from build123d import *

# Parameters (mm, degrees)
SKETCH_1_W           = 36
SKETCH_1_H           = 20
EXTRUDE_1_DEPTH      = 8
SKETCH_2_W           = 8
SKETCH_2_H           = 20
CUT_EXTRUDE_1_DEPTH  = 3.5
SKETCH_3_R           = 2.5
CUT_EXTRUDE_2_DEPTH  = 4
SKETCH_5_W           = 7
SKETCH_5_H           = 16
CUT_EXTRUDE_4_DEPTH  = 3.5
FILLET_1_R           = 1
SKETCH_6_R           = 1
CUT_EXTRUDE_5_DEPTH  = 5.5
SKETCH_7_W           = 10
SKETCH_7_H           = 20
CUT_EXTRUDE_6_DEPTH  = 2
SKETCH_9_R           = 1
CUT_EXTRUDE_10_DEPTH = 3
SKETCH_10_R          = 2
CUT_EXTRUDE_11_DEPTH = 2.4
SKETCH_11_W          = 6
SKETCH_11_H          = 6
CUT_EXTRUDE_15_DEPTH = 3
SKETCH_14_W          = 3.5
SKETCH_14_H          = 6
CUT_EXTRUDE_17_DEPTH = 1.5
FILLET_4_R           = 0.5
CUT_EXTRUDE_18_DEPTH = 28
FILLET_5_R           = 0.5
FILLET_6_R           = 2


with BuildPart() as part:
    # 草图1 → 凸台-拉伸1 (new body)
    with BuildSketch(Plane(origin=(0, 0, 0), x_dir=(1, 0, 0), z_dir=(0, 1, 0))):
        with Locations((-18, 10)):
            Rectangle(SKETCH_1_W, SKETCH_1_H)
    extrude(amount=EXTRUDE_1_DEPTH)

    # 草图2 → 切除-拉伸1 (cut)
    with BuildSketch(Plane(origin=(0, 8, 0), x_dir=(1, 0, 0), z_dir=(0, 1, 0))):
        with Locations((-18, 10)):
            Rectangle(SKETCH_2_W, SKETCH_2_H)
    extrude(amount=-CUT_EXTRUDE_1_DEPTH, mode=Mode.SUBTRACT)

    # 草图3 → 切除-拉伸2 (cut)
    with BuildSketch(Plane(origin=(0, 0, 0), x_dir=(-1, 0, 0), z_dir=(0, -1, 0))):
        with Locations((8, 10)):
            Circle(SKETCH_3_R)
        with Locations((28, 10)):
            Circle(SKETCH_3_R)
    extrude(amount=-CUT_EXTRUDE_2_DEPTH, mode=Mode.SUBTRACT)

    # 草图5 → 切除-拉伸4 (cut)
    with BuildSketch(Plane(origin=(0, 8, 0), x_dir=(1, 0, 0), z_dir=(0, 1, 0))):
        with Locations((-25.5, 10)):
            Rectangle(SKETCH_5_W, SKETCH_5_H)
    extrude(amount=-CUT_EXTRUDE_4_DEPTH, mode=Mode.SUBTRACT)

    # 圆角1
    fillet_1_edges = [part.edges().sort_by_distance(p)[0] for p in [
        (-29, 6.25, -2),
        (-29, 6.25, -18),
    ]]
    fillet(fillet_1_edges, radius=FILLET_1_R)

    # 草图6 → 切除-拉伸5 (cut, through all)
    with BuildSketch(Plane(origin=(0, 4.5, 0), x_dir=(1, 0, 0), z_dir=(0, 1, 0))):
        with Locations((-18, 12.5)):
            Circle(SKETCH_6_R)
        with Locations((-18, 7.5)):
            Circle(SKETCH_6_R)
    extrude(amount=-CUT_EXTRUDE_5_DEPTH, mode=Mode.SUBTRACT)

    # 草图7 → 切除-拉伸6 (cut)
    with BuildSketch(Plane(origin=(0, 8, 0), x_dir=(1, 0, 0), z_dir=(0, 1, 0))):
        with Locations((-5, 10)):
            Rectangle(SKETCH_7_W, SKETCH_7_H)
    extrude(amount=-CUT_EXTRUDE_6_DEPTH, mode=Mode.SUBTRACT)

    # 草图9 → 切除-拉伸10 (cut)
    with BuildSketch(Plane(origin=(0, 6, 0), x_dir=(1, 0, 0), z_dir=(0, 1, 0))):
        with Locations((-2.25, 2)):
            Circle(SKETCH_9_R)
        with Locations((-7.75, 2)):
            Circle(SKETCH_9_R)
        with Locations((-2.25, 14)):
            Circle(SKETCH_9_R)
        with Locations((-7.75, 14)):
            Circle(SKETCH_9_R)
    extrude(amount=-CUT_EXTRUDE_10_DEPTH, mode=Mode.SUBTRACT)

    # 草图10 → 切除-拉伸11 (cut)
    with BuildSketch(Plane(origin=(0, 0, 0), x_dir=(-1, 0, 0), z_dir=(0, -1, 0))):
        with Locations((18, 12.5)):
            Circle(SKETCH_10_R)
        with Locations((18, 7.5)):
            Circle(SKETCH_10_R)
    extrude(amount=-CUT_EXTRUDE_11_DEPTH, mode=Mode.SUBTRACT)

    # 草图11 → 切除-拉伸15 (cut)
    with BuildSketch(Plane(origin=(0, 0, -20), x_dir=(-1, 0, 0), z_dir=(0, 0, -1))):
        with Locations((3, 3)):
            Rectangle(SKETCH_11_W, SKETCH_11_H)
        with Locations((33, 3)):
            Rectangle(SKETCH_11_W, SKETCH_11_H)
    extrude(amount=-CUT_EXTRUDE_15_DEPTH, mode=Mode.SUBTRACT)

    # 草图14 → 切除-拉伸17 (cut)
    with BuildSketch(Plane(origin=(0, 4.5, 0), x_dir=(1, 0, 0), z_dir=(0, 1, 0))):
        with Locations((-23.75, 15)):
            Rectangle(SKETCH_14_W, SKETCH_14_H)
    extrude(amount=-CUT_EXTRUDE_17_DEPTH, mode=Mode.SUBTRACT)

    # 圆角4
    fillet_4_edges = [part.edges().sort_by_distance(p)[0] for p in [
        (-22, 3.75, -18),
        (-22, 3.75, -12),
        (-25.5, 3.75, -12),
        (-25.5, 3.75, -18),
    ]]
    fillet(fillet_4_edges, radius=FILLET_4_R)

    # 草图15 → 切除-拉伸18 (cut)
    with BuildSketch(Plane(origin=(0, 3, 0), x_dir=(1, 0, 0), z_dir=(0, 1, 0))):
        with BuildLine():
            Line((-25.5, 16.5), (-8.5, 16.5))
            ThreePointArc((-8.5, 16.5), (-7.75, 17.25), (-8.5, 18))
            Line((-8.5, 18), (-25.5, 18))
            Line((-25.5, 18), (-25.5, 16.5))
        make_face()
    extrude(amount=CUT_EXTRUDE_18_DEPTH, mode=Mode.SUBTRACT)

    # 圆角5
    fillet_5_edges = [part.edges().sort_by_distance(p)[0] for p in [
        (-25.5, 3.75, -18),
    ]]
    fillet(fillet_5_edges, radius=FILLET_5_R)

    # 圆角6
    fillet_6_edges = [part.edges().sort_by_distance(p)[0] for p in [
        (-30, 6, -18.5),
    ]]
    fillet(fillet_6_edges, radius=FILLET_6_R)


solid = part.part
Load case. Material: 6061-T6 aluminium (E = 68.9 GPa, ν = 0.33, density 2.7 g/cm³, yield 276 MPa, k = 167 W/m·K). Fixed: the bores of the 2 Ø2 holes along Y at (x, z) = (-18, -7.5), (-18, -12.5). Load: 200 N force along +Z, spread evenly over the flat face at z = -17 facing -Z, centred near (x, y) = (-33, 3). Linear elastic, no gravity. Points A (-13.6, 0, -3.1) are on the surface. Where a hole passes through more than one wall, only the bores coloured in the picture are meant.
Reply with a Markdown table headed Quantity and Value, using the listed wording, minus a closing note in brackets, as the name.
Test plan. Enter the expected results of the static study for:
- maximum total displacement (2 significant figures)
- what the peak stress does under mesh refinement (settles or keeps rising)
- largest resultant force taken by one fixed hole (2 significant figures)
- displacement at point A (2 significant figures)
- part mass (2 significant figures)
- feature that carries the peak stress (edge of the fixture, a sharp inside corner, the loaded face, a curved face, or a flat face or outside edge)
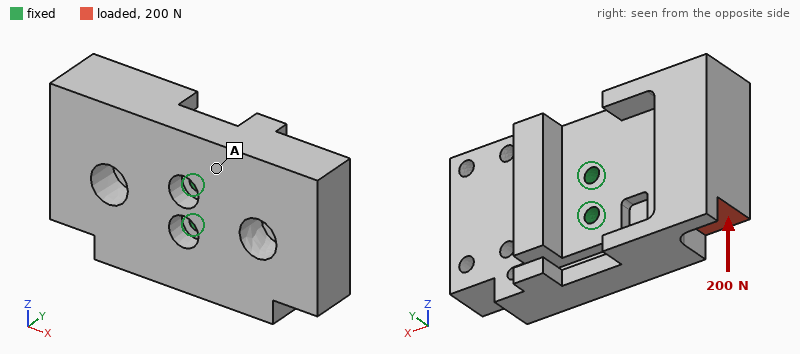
| Quantity | Value |
|---|---|
| maximum total displacement | 14 µm |
| what the peak stress does under mesh refinement | keeps rising |
| largest resultant force taken by one fixed hole | 470 N |
| displacement at point A | 4.0 µm |
| part mass | 10 g |
| feature that carries the peak stress | edge of the fixture |
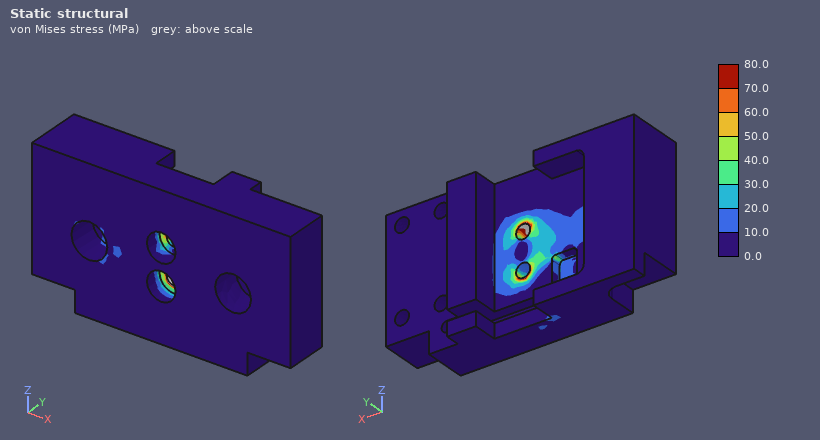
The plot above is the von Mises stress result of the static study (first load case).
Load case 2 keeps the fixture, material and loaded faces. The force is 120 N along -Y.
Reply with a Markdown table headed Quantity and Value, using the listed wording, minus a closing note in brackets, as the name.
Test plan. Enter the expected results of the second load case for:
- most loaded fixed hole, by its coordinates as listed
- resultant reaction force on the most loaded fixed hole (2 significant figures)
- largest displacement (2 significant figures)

| Quantity | Value |
|---|---|
| most loaded fixed hole, by its coordinates as listed | (-18, -12.5) |
| resultant reaction force on the most loaded fixed hole | 170 N |
| largest displacement | 61 µm |
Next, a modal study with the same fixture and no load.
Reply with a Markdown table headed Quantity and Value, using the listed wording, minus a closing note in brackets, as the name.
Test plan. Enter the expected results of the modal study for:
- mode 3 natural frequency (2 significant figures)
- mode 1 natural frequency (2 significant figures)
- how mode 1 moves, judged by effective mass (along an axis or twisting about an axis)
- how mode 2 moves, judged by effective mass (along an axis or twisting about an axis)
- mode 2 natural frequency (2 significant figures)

| Quantity | Value |
|---|---|
| mode 3 natural frequency | 9200 Hz |
| mode 1 natural frequency | 4200 Hz |
| how mode 1 moves, judged by effective mass | twisting about Z |
| how mode 2 moves, judged by effective mass | along Y |
| mode 2 natural frequency | 8800 Hz |
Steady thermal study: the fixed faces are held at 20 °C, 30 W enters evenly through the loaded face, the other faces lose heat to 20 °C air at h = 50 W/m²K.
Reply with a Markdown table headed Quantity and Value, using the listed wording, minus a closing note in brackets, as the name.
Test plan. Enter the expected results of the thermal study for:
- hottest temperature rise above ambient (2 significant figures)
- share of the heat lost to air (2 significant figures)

| Quantity | Value |
|---|---|
| hottest temperature rise above ambient | 57 K |
| share of the heat lost to air | 7.4 % |
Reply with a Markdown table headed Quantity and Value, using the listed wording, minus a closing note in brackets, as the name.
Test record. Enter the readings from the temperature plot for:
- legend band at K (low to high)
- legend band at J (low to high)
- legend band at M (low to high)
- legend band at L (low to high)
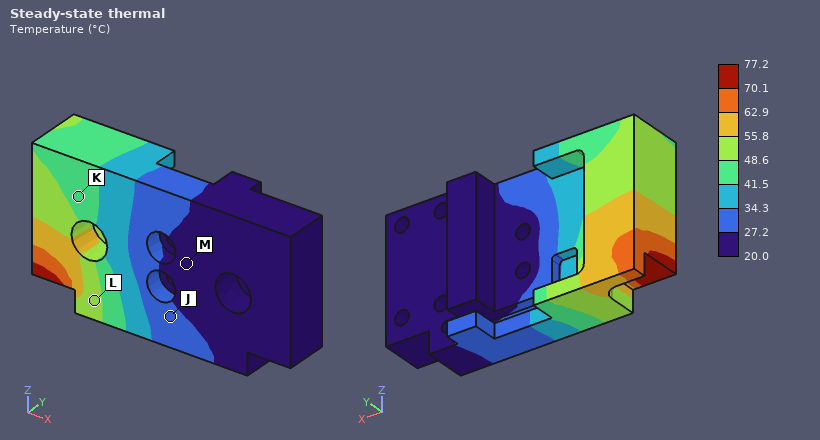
| Quantity | Value |
|---|---|
| legend band at K | 41.5 to 48.6 °C |
| legend band at J | 27.2 to 34.3 °C |
| legend band at M | 20.0 to 27.2 °C |
| legend band at L | 48.6 to 55.8 °C |
